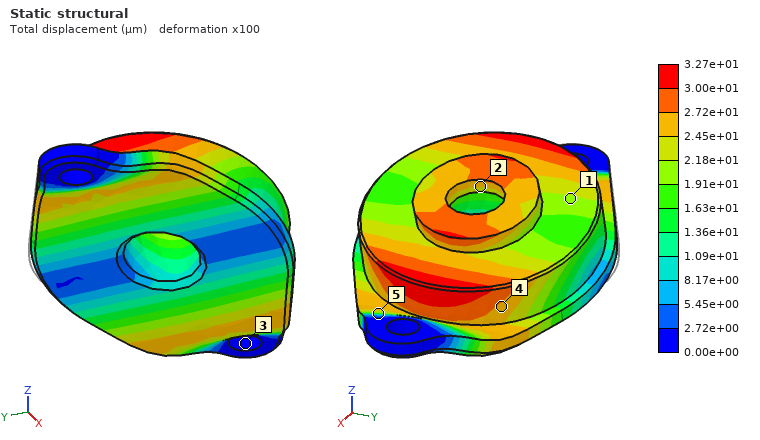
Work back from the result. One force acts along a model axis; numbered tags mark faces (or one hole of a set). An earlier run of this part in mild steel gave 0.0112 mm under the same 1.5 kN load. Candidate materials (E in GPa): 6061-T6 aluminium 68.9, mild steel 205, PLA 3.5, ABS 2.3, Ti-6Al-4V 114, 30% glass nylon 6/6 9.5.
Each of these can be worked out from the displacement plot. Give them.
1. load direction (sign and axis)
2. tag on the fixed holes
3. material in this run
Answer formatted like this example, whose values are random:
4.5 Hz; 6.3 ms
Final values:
+X; 3; 6061-T6 aluminium
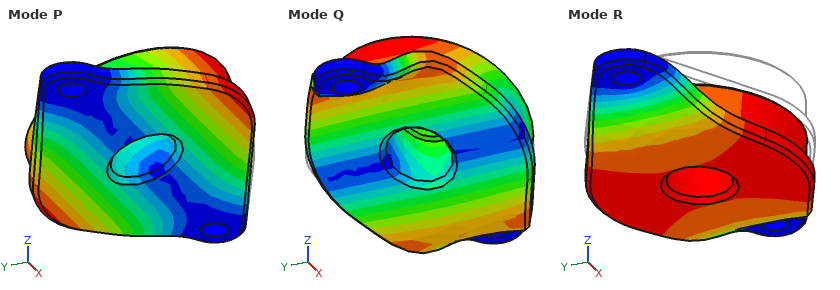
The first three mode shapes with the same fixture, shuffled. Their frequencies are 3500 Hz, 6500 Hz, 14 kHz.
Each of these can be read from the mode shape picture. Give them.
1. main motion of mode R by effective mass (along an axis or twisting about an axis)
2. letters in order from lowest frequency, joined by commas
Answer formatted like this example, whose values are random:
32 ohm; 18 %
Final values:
along Z; P, R, Q
